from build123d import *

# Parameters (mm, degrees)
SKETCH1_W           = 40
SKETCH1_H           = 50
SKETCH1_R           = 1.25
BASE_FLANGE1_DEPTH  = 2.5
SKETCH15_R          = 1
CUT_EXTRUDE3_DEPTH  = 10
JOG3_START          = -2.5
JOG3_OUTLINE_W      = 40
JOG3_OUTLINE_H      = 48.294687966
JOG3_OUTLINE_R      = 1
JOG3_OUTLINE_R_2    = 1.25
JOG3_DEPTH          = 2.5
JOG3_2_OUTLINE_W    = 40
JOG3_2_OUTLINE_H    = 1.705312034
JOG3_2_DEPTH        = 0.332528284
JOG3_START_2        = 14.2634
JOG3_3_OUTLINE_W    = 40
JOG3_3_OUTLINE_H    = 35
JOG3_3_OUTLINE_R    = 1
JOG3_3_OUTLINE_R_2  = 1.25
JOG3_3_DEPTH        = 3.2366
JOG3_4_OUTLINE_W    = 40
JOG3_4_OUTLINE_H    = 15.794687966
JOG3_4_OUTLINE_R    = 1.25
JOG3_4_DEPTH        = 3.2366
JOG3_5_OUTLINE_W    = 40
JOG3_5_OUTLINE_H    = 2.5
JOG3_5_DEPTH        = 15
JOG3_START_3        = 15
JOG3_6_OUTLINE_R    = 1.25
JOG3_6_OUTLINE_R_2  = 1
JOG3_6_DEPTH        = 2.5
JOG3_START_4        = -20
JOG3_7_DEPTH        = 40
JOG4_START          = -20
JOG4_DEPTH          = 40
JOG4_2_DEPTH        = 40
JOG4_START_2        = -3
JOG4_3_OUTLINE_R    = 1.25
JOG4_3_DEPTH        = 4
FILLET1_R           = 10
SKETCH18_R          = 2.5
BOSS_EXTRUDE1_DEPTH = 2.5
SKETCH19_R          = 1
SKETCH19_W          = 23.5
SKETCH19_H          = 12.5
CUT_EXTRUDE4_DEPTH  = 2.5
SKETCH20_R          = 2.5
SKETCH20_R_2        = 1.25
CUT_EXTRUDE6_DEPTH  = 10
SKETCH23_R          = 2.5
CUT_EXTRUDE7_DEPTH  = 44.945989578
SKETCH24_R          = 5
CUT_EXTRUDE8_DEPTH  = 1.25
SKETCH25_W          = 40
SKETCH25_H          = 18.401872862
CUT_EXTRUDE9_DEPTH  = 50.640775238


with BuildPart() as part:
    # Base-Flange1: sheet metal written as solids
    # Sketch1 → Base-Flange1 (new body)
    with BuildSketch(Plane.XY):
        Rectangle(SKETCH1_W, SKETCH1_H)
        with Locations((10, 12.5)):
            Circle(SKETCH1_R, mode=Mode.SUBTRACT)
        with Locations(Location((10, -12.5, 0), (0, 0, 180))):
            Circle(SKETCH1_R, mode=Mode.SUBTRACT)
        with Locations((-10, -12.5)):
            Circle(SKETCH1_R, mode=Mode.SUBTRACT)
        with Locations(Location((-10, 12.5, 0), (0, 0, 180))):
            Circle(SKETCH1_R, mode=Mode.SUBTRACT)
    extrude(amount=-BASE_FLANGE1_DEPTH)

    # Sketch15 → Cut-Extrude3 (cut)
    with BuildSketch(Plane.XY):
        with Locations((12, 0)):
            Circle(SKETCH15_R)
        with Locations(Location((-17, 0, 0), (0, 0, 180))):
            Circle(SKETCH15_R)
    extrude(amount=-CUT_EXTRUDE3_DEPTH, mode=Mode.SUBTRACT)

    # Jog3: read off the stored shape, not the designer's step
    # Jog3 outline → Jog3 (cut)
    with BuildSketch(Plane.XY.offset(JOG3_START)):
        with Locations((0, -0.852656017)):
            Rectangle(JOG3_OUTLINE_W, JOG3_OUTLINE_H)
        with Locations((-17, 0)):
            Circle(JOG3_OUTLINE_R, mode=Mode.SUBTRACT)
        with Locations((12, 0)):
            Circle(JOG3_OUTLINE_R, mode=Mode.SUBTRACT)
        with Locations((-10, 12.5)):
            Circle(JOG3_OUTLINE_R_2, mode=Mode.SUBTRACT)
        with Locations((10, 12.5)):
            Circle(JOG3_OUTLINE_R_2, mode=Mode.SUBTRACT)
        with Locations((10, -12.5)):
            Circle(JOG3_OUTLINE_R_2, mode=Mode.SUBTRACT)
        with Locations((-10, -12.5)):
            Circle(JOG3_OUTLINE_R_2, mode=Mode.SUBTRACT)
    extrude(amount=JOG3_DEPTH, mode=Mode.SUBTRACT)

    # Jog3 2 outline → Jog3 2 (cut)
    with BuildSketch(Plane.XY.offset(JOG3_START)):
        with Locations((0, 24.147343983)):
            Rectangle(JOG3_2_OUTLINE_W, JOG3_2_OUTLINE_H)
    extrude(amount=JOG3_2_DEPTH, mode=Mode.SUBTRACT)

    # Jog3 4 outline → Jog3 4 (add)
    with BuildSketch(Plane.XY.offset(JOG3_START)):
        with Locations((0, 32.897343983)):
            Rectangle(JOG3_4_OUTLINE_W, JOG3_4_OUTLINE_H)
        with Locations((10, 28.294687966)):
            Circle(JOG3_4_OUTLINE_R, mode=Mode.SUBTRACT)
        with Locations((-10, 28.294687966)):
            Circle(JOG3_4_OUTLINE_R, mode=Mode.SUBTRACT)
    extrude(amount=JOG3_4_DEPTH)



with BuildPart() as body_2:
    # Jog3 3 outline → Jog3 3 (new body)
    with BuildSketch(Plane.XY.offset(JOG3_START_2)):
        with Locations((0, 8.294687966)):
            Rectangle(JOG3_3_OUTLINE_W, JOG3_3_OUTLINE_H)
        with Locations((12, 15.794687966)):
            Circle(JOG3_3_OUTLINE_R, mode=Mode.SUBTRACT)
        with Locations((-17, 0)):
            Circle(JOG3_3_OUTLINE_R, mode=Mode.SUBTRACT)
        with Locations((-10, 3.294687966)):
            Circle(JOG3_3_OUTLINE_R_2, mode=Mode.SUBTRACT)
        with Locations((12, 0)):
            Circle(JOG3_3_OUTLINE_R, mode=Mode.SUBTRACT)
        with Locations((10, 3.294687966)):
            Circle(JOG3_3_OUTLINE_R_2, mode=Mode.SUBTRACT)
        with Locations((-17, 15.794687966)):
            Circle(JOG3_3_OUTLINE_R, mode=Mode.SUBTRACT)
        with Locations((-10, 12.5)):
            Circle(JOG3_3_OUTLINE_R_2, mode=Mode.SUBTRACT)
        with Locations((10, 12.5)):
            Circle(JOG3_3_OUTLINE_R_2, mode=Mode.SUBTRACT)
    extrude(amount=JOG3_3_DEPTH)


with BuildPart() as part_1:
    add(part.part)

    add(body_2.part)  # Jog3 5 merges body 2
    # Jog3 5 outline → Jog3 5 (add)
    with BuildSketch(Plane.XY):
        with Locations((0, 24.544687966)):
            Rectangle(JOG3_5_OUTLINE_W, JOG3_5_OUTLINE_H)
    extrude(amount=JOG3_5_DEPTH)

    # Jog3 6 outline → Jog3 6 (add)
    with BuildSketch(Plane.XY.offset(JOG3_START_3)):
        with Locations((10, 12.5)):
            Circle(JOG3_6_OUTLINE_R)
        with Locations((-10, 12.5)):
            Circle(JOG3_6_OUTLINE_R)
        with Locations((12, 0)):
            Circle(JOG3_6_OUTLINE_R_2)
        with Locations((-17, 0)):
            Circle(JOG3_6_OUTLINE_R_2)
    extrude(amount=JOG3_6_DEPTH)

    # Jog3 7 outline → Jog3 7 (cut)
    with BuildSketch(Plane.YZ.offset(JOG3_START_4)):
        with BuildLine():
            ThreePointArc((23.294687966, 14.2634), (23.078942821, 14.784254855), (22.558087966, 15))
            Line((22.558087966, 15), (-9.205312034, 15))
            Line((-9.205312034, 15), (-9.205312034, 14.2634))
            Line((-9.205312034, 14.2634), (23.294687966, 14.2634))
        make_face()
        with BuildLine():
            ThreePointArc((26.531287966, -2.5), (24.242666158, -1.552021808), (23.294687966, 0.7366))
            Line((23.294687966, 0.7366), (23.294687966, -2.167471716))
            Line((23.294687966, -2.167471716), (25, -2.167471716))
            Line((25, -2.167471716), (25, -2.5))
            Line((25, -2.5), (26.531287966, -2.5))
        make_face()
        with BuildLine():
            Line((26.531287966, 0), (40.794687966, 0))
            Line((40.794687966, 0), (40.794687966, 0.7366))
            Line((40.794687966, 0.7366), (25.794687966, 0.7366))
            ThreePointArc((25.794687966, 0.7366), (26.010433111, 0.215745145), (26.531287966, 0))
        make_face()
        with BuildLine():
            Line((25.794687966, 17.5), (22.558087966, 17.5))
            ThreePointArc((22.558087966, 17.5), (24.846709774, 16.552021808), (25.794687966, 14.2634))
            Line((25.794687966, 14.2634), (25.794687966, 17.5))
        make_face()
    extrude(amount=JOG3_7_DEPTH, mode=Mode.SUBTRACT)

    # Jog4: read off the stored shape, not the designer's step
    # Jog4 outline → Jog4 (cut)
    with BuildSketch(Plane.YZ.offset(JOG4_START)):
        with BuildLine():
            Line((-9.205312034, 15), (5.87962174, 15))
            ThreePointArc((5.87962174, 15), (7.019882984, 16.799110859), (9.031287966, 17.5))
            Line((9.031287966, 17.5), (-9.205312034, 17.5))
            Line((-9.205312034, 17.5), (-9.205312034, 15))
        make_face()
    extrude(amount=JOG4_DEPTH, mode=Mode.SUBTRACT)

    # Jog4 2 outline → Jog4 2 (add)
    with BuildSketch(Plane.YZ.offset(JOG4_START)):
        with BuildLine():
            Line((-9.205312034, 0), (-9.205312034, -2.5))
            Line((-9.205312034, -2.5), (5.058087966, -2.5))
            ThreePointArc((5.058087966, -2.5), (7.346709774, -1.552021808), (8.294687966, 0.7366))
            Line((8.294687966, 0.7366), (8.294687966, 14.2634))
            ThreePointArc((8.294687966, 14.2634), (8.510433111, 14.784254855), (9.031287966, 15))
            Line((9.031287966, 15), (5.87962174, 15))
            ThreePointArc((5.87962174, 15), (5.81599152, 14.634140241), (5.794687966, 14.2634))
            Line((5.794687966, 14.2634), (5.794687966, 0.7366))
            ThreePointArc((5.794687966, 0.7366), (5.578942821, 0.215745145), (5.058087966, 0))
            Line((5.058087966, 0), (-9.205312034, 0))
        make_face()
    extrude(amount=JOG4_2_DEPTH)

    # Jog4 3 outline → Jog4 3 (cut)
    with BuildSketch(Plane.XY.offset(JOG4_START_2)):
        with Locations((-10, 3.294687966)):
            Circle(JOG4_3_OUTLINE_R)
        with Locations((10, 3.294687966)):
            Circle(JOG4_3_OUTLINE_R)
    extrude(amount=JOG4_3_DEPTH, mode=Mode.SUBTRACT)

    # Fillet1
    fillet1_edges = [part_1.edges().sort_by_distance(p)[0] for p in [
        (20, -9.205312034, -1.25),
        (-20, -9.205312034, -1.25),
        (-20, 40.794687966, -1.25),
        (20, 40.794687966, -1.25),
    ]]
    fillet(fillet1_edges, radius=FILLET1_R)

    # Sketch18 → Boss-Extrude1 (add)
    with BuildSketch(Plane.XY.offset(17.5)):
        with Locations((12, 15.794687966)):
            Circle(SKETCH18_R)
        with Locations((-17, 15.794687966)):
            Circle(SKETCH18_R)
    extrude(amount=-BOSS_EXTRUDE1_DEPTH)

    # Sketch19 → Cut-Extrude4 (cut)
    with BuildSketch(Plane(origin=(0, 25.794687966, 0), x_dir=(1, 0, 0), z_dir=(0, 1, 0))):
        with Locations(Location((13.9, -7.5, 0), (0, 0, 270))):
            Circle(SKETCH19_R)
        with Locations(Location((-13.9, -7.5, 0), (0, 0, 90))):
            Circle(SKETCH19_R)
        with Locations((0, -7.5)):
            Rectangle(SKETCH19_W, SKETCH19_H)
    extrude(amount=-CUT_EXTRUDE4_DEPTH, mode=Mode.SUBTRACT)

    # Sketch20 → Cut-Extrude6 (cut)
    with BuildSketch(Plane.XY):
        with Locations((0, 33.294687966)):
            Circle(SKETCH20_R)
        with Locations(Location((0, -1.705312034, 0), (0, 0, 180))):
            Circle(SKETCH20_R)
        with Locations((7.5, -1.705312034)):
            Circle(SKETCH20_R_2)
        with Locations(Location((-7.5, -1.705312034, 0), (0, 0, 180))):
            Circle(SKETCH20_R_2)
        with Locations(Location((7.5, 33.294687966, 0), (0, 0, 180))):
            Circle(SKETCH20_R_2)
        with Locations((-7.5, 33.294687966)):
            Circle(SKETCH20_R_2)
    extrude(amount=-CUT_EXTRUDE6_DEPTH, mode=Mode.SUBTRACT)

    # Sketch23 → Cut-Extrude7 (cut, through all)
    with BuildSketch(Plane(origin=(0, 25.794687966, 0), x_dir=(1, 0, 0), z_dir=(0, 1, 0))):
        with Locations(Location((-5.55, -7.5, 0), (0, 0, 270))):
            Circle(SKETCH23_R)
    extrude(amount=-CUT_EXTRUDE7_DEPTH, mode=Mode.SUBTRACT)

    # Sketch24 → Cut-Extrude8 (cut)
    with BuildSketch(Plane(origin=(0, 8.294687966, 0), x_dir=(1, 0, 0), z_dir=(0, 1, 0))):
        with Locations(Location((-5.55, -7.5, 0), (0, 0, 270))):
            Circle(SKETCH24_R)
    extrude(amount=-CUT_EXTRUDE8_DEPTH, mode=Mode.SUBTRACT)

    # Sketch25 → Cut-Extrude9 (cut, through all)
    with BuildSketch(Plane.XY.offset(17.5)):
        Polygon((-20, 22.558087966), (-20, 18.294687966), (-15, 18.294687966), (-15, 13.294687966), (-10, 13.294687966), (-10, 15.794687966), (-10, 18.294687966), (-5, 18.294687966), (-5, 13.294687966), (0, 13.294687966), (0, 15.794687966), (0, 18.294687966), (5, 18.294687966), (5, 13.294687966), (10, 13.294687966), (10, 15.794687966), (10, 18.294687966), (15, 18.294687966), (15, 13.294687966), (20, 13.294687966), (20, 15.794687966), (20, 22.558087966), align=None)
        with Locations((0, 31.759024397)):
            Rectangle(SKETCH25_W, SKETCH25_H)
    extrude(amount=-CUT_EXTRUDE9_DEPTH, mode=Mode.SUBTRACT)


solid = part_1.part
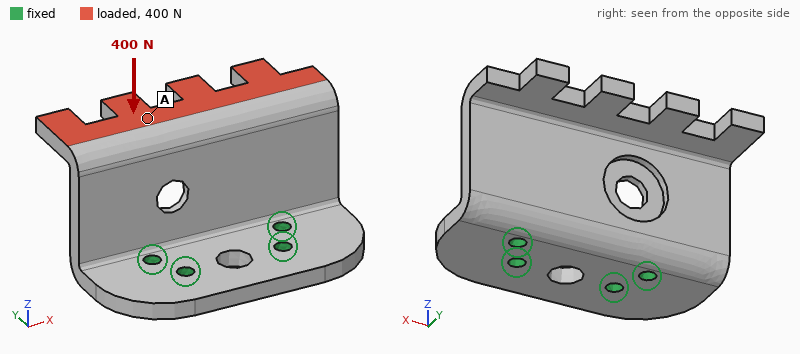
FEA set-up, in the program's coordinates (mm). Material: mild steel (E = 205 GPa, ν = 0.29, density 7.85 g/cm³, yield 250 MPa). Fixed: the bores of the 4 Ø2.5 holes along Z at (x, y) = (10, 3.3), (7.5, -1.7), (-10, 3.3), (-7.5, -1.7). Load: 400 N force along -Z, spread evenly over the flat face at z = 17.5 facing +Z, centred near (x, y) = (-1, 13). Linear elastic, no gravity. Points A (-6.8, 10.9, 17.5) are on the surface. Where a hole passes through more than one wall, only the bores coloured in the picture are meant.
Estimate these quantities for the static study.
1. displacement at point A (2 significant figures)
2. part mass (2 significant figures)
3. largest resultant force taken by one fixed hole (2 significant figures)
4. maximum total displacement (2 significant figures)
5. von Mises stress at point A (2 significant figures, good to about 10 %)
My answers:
0.071 mm
29 g
320 N
0.10 mm
24 MPa
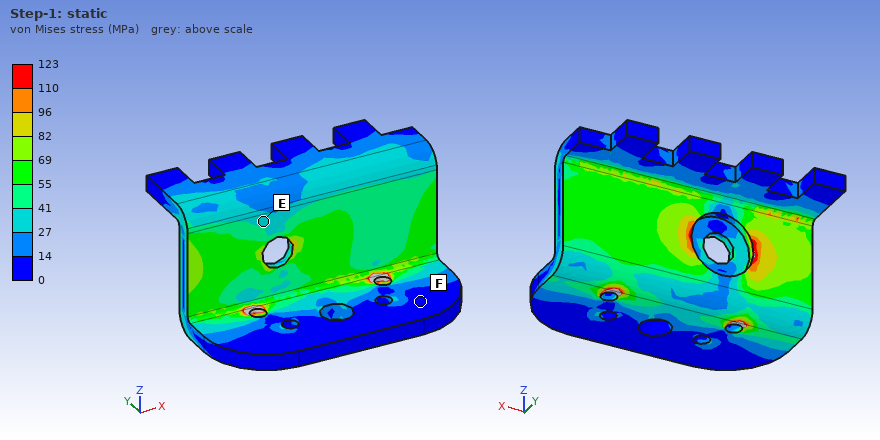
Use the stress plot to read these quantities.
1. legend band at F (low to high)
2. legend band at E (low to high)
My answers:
0 to 14 MPa
27 to 41 MPa
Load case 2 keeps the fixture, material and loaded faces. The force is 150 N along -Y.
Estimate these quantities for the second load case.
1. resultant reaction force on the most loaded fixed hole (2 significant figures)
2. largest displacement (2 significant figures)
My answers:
110 N
71 µm
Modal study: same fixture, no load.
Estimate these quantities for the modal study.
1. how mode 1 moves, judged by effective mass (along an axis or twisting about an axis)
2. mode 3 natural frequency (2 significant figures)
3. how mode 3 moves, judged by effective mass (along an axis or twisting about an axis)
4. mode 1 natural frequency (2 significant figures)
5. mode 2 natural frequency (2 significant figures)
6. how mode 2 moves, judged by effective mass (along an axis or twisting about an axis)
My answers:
along Y
11 kHz
along X
2800 Hz
4900 Hz
twisting about Z
